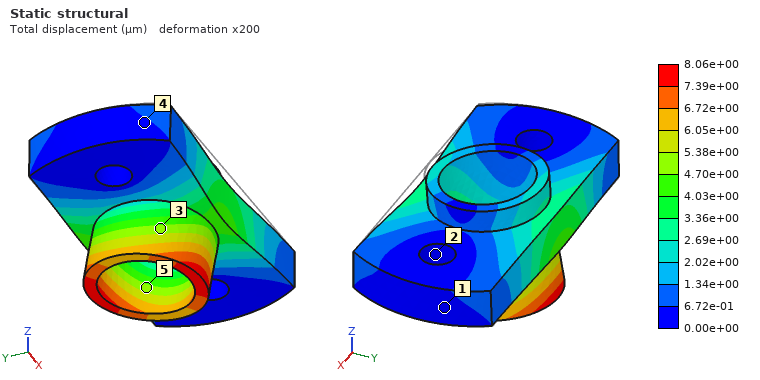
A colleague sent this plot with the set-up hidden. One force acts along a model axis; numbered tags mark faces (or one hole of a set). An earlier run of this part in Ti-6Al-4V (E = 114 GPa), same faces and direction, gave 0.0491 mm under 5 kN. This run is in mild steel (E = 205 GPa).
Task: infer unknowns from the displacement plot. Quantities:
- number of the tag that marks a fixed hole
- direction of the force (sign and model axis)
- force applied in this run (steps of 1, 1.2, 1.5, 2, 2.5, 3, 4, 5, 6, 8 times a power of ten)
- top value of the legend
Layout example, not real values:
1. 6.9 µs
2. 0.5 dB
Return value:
1. 2
2. +Y
3. 1.5 kN
4. 8.06e+00 µm
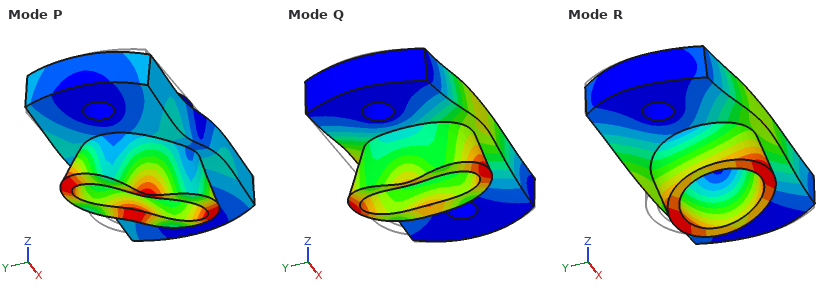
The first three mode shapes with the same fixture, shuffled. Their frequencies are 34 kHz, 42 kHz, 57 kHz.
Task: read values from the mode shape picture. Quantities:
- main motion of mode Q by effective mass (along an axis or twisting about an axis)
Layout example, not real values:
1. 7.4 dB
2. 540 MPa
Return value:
1. along Z
